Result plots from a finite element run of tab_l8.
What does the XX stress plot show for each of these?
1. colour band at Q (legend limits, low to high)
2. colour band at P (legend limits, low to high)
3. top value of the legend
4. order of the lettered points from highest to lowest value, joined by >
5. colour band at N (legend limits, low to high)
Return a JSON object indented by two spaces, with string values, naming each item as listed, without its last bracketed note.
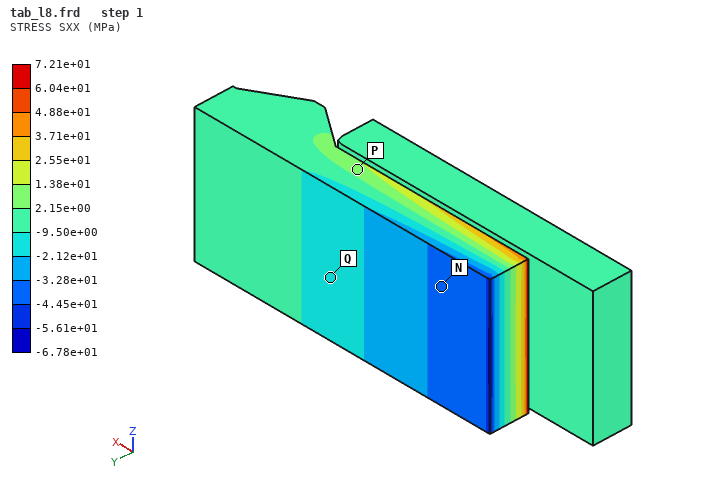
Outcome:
{
  "colour band at Q": "-2.12e+01 to -9.50e+00 MPa",
  "colour band at P": "2.15e+00 to 1.38e+01 MPa",
  "top value of the legend": "7.21e+01 MPa",
  "order of the lettered points from highest to lowest value, joined by >": "P > Q > N",
  "colour band at N": "-4.45e+01 to -3.28e+01 MPa"
}
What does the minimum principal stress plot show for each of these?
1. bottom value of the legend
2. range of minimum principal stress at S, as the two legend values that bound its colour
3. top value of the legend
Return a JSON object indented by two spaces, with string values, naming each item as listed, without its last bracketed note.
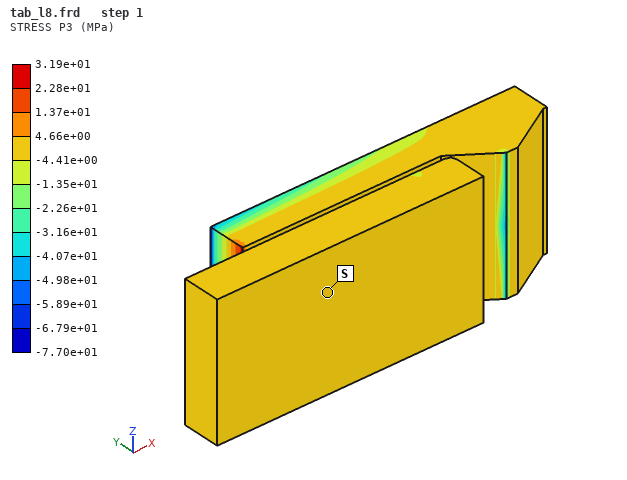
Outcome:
{
  "bottom value of the legend": "-7.70e+01 MPa",
  "range of minimum principal stress at S, as the two legend values that bound its colour": "-4.41e+00 to 4.66e+00 MPa",
  "top value of the legend": "3.19e+01 MPa"
}
